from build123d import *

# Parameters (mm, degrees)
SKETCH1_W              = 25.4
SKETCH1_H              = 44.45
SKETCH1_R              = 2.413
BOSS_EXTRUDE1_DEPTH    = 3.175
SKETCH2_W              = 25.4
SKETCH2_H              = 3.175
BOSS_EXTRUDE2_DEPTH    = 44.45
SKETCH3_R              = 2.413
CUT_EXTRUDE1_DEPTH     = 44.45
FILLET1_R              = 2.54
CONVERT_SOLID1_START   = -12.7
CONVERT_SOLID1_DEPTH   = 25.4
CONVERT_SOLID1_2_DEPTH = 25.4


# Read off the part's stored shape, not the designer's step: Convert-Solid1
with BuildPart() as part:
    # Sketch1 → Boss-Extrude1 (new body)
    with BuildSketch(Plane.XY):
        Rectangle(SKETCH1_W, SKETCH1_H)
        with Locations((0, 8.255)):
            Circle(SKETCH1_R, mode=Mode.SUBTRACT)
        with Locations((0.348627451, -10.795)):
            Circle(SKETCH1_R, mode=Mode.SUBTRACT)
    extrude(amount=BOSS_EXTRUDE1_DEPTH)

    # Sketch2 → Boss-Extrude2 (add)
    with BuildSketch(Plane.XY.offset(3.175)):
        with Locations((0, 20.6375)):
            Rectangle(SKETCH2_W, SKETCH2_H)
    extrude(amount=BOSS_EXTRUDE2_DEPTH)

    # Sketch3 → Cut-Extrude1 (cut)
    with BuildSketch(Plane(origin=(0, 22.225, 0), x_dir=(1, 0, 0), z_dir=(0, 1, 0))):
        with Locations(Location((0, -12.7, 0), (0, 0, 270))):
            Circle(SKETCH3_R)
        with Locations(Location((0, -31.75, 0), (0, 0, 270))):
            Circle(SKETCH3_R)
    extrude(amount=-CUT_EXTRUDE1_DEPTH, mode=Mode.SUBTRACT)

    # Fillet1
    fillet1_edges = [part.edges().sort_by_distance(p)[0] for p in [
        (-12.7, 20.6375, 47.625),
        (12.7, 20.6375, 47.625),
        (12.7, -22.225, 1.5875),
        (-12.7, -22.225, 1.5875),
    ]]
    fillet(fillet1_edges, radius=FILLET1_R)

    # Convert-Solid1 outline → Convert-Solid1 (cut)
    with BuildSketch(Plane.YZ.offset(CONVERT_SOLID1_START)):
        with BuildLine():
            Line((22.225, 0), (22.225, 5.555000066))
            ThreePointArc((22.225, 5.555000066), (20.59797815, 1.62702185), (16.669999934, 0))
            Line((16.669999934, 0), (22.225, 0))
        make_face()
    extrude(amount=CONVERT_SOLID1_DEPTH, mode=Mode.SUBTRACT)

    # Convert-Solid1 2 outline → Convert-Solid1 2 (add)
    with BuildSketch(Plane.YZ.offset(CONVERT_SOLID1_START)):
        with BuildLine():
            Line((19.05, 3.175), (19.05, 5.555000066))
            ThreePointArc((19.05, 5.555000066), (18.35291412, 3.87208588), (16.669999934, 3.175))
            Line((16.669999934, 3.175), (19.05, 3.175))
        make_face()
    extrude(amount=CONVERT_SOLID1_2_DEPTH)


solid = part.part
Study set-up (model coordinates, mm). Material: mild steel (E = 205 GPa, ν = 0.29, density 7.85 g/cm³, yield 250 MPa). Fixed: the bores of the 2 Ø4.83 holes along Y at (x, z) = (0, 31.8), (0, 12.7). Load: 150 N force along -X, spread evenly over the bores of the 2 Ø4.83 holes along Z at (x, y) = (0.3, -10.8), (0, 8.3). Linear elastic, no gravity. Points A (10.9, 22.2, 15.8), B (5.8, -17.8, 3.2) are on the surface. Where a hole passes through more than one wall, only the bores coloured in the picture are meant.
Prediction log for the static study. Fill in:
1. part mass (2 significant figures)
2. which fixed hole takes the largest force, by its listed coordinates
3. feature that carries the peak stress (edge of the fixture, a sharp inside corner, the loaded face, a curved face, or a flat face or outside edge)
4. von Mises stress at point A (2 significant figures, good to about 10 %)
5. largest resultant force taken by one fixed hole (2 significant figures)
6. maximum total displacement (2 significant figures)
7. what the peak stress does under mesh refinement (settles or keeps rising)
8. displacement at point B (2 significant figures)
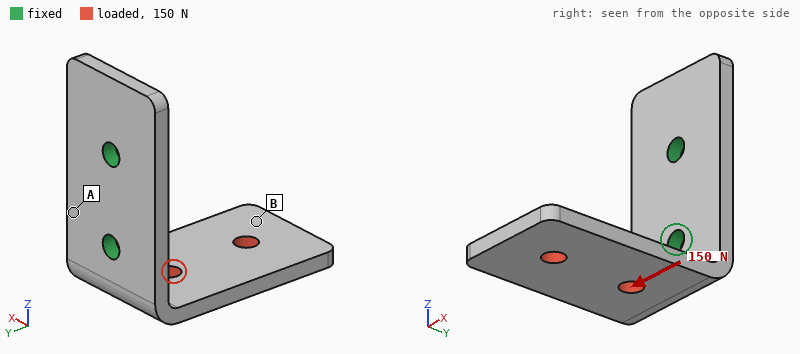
53 g
(0, 12.7)
edge of the fixture
29 MPa
210 N
59 µm
keeps rising
52 µm
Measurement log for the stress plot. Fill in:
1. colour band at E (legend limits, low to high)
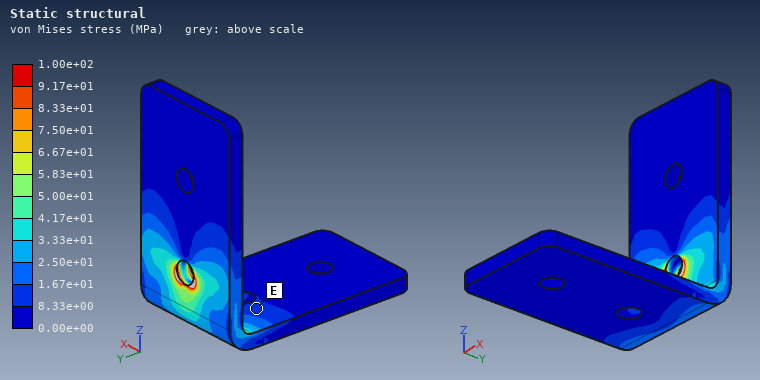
8.33e+00 to 1.67e+01 MPa
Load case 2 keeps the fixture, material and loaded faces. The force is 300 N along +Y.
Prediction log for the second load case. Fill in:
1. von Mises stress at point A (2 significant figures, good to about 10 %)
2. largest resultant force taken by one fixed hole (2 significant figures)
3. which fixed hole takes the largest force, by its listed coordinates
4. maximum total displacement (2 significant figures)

17 MPa
340 N
(0, 12.7)
56 µm
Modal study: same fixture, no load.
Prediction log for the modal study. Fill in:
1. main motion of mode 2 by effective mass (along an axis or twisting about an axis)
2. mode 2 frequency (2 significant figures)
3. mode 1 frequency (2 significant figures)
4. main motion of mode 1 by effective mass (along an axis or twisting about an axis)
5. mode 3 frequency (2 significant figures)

along X
1900 Hz
1100 Hz
along Z
4800 Hz
